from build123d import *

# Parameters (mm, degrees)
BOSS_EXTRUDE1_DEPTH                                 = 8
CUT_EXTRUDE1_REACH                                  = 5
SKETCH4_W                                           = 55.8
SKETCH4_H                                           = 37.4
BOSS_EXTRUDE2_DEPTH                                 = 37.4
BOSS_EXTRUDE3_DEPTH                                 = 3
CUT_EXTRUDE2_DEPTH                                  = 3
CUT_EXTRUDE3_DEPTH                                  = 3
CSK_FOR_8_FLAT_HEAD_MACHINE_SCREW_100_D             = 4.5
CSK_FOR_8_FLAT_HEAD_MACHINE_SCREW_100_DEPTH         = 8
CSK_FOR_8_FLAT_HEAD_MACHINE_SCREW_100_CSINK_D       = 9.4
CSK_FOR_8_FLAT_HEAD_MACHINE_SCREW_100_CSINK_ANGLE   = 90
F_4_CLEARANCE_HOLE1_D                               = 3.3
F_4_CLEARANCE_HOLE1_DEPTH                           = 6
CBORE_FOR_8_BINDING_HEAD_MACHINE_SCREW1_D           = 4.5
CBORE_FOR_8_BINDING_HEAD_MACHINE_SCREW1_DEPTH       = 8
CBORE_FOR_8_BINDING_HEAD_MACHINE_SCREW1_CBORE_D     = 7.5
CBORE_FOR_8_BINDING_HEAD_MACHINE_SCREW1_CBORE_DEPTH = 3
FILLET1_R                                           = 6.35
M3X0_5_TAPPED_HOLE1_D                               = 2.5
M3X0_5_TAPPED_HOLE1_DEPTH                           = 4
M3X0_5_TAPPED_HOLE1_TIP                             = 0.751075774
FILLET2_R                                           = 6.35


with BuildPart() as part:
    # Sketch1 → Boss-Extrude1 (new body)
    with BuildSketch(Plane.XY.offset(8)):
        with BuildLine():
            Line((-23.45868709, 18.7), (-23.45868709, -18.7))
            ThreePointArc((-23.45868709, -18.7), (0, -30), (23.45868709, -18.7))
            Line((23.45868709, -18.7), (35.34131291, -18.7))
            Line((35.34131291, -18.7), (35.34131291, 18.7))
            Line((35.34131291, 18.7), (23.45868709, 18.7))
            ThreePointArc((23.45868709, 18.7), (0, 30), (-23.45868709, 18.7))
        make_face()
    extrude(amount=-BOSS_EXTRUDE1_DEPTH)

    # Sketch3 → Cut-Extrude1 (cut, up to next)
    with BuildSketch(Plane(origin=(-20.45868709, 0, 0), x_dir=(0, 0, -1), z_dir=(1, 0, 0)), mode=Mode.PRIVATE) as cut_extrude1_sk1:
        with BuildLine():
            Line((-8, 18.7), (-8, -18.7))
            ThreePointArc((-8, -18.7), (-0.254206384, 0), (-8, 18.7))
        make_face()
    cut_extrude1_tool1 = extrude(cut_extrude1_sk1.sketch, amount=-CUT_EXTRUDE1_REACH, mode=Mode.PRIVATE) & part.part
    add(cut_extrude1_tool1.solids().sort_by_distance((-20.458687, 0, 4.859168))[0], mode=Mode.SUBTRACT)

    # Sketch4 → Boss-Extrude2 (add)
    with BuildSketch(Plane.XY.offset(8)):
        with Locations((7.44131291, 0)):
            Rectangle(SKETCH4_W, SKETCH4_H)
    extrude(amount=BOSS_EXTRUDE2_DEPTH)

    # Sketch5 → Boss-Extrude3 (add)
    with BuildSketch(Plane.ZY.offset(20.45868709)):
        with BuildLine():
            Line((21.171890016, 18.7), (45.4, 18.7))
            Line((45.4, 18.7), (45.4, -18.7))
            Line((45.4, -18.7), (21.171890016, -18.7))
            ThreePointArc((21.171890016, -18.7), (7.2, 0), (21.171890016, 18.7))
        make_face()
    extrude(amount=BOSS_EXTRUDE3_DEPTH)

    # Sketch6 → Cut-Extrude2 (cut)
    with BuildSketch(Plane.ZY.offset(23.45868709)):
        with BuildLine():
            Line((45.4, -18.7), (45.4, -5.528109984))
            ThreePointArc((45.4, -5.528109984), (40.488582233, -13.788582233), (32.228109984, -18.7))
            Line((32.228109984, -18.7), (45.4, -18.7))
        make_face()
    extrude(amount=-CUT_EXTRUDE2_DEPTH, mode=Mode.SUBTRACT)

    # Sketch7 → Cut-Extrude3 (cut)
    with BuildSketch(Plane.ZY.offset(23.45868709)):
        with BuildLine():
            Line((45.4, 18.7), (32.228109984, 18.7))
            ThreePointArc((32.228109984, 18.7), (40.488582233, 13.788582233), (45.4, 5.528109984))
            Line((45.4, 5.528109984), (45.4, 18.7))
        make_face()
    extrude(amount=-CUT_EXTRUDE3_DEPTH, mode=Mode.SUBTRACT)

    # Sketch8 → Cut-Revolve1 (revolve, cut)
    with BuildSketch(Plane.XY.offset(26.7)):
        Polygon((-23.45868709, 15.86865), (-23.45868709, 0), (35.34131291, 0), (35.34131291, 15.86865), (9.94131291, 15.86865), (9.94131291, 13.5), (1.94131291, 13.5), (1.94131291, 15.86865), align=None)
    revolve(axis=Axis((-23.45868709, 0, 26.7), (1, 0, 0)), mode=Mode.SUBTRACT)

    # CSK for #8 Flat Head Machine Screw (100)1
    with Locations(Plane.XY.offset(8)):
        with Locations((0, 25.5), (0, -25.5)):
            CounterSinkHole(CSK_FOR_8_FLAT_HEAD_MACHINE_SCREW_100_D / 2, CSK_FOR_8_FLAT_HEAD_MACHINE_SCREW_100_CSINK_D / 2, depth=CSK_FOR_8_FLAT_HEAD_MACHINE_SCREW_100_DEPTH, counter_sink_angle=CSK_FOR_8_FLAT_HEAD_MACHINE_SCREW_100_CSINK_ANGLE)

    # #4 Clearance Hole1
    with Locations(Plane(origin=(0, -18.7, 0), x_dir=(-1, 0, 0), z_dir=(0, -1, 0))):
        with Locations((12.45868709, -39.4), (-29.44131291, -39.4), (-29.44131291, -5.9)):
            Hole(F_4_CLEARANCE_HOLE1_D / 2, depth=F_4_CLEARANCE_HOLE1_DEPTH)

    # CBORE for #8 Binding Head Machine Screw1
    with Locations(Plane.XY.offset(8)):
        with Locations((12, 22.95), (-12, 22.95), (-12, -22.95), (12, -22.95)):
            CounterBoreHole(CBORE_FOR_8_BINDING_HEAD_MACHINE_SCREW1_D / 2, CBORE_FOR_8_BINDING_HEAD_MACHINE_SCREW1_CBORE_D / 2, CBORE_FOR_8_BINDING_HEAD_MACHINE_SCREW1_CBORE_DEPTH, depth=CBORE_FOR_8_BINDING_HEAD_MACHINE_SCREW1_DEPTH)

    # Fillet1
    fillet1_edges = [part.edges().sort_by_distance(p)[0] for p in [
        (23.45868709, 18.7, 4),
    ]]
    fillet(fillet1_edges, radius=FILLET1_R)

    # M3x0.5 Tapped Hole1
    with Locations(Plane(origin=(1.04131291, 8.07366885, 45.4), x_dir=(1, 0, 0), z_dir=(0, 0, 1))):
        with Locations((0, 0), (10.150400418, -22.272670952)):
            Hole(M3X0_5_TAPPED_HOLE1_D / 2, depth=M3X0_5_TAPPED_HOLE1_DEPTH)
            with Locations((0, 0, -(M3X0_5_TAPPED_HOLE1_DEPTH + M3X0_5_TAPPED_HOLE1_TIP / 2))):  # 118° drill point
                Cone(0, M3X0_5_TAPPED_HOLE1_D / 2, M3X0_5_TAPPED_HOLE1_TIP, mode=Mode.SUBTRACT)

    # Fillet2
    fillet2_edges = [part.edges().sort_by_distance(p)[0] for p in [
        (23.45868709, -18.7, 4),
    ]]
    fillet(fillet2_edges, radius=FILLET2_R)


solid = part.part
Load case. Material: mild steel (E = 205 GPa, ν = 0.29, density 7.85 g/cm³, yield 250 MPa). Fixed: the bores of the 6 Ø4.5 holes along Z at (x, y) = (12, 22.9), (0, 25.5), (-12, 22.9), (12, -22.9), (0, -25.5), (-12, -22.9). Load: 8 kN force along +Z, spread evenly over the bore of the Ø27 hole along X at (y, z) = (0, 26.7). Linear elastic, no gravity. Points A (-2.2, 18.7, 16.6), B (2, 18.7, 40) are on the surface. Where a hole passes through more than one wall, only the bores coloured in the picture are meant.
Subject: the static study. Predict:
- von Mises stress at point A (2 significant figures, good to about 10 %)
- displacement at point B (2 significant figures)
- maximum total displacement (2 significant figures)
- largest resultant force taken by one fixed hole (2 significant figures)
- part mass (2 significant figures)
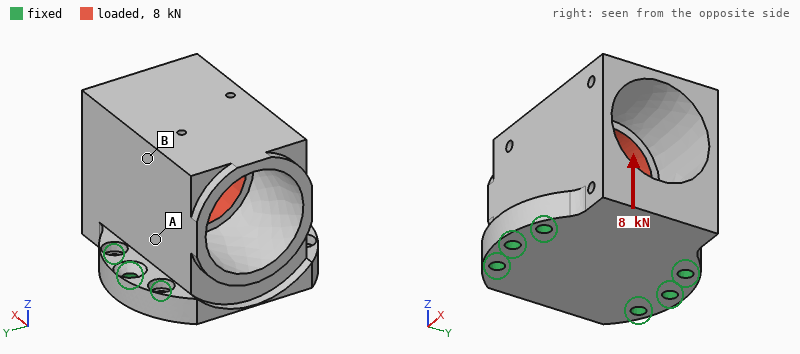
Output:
26 MPa
5.8 µm
11 µm
2.6 kN
460 g
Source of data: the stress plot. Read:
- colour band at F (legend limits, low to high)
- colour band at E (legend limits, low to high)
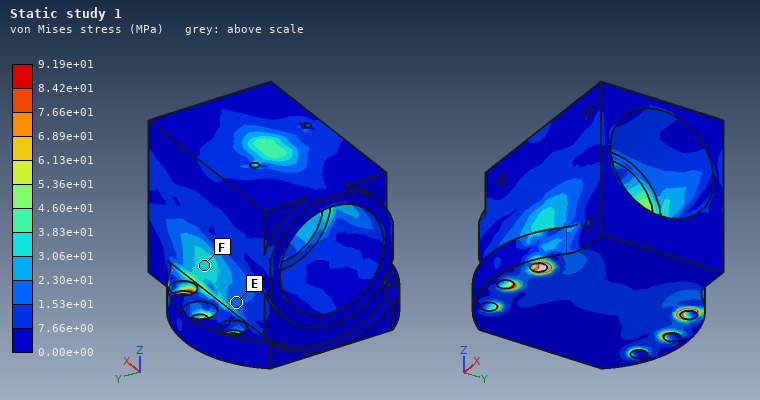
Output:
3.06e+01 to 3.83e+01 MPa
1.53e+01 to 2.30e+01 MPa
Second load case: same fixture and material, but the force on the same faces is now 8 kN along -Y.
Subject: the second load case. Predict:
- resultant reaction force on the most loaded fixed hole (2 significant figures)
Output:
2.6 kN
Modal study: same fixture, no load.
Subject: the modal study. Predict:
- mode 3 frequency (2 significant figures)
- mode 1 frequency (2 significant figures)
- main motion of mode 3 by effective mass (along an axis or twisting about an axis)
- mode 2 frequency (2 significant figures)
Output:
8400 Hz
4800 Hz
twisting about Z
4900 Hz
